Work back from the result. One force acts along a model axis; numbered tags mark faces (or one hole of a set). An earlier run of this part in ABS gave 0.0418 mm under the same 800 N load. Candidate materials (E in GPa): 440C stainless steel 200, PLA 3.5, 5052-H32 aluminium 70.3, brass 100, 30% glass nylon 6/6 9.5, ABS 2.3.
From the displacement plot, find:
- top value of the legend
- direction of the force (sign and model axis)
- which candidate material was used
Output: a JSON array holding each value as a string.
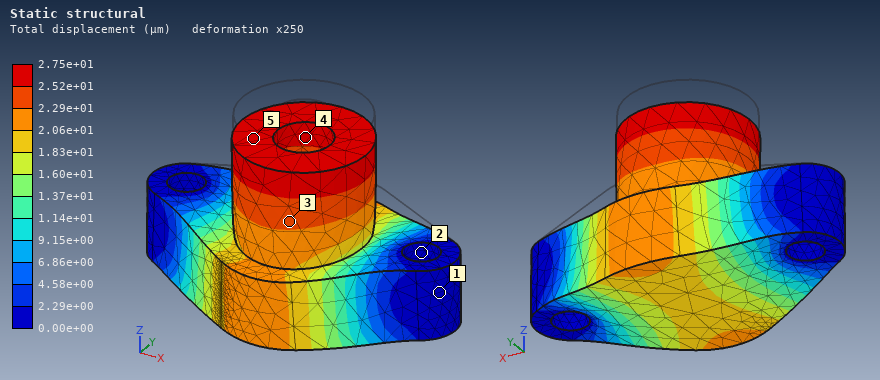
["2.75e+01 µm", "-Z", "PLA"]
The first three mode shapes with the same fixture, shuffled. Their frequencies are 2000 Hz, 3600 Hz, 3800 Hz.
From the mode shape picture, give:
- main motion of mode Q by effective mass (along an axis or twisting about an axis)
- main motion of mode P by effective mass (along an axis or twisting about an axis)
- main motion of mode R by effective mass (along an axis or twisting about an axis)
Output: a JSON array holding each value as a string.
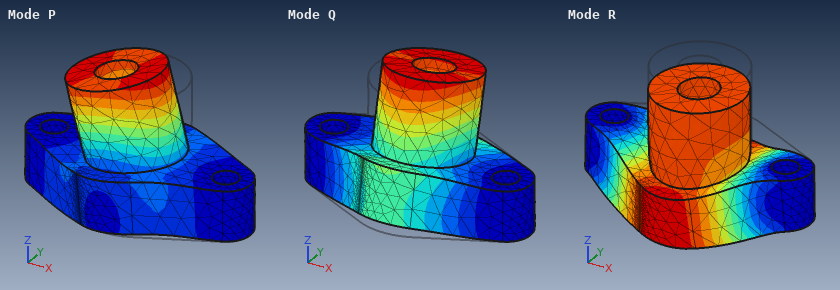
["along Y", "along X", "along Z"]
